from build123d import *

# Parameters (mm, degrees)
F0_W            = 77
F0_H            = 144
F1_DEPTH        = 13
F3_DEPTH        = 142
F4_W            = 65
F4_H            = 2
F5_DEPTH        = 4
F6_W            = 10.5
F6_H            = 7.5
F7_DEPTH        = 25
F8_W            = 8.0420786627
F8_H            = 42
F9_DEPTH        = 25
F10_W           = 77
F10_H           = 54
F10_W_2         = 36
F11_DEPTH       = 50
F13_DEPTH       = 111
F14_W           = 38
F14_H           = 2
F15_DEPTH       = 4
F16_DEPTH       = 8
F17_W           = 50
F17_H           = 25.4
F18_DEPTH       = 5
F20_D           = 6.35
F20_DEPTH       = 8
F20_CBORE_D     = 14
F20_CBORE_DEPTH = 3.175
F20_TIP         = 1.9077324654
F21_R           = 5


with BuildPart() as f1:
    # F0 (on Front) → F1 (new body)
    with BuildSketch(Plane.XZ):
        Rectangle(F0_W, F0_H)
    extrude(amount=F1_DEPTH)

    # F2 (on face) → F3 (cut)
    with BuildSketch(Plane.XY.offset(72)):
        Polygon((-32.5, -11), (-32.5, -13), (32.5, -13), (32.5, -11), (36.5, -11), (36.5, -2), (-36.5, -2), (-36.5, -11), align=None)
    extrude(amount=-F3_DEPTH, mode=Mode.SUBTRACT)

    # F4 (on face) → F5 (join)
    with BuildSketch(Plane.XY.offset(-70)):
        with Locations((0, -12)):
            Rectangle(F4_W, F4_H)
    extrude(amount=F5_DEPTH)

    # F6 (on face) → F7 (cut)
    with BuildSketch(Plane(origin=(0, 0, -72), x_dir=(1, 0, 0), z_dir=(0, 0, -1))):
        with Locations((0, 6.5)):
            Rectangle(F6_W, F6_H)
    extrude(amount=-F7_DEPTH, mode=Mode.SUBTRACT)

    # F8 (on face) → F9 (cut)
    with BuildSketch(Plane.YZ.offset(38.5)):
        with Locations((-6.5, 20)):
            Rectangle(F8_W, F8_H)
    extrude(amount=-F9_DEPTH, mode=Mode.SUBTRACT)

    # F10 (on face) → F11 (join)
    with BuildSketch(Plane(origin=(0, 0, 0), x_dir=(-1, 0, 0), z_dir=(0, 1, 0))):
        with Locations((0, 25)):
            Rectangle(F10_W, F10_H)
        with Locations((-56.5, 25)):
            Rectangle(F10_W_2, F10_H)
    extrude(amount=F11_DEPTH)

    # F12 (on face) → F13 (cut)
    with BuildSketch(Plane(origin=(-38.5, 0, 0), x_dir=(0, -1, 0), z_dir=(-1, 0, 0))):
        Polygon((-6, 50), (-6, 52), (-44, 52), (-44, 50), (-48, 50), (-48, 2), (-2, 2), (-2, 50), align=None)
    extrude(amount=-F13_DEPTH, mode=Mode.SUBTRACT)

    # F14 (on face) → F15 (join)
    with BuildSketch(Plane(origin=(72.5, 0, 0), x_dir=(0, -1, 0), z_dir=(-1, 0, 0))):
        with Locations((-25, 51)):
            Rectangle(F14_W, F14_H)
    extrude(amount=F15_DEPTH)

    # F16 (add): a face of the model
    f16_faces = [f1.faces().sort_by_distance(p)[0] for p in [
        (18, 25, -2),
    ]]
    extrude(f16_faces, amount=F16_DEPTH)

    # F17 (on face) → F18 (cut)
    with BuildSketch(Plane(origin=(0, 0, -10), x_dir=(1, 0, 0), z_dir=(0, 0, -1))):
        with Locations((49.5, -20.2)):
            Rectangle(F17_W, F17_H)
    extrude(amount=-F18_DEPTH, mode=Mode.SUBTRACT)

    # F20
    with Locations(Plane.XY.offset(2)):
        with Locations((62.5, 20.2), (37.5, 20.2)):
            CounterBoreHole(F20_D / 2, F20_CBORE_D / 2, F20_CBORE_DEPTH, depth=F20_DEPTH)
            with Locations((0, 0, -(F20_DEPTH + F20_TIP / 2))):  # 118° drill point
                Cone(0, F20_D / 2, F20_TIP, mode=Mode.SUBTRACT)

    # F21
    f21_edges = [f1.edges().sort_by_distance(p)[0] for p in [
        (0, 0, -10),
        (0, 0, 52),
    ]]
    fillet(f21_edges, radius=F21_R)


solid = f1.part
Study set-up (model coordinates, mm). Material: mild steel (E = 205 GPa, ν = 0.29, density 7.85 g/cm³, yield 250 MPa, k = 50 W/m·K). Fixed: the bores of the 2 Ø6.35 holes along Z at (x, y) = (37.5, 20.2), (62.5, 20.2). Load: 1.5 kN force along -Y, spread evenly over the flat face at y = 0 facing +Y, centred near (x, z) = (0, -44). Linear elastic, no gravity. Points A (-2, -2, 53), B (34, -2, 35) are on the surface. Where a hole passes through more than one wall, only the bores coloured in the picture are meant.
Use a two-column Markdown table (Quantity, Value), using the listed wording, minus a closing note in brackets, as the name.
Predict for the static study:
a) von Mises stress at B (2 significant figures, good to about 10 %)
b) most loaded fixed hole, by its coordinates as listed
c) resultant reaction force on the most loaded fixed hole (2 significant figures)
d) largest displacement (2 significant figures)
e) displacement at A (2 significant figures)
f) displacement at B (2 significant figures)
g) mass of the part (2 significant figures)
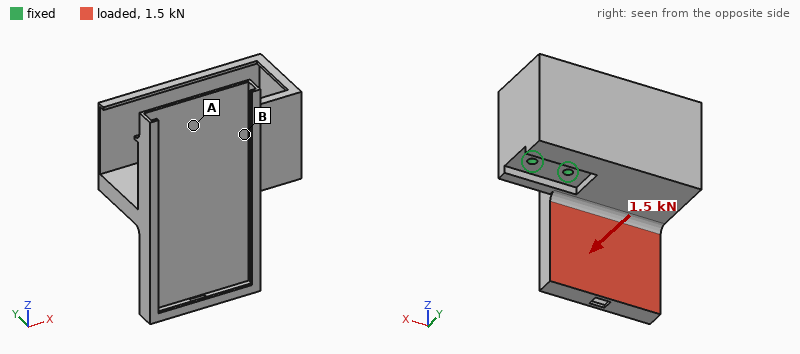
| Quantity | Value |
|---|---|
| von Mises stress at B | 41 MPa |
| most loaded fixed hole, by its coordinates as listed | (37.5, 20.2) |
| resultant reaction force on the most loaded fixed hole | 3.4 kN |
| largest displacement | 0.52 mm |
| displacement at A | 0.23 mm |
| displacement at B | 0.13 mm |
| mass of the part | 960 g |
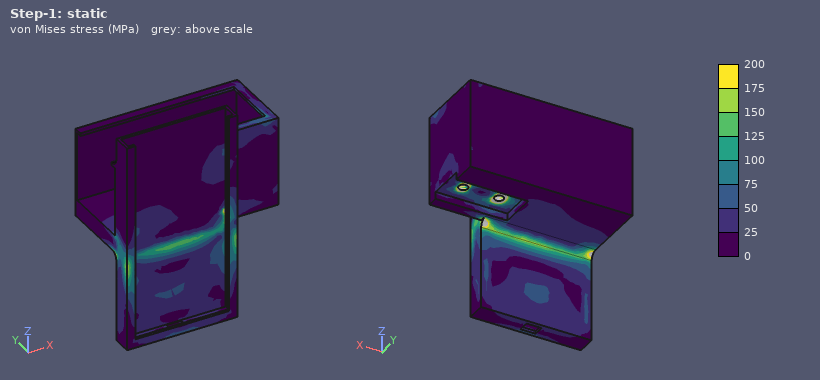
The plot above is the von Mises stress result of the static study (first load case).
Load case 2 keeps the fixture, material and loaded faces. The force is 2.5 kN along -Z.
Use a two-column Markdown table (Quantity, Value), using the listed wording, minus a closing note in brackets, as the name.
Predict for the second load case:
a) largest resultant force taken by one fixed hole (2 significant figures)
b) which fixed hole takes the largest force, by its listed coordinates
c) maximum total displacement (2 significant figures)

| Quantity | Value |
|---|---|
| largest resultant force taken by one fixed hole | 5.3 kN |
| which fixed hole takes the largest force, by its listed coordinates | (37.5, 20.2) |
| maximum total displacement | 0.30 mm |
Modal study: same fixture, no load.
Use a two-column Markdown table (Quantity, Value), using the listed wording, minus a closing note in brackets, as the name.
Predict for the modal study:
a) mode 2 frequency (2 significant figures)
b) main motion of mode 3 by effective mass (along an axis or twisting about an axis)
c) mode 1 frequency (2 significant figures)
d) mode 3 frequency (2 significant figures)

| Quantity | Value |
|---|---|
| mode 2 frequency | 780 Hz |
| main motion of mode 3 by effective mass | along Z |
| mode 1 frequency | 600 Hz |
| mode 3 frequency | 970 Hz |
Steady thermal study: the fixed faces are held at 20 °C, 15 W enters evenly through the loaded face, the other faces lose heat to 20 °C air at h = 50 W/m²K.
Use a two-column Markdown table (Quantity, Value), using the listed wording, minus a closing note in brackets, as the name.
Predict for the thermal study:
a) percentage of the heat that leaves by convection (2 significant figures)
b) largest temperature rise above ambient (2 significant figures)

| Quantity | Value |
|---|---|
| percentage of the heat that leaves by convection | 86 % |
| largest temperature rise above ambient | 23 K |
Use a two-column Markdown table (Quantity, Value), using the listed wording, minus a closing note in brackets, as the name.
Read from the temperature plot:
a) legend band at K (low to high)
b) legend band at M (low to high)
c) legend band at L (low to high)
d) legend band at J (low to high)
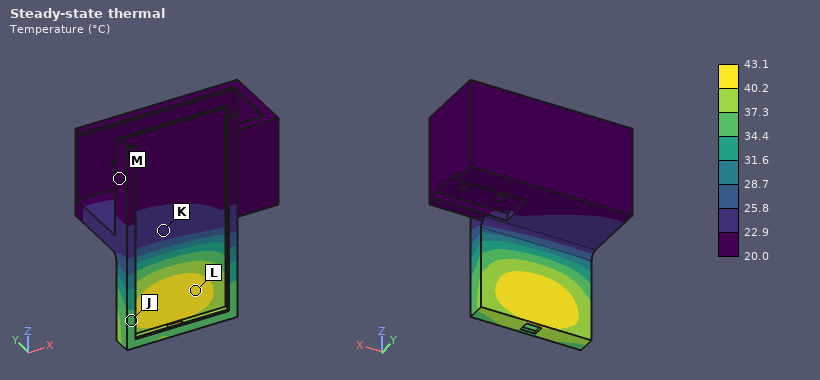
| Quantity | Value |
|---|---|
| legend band at K | 22.9 to 25.8 °C |
| legend band at M | 20.0 to 22.9 °C |
| legend band at L | 40.2 to 43.1 °C |
| legend band at J | 34.4 to 37.3 °C |
